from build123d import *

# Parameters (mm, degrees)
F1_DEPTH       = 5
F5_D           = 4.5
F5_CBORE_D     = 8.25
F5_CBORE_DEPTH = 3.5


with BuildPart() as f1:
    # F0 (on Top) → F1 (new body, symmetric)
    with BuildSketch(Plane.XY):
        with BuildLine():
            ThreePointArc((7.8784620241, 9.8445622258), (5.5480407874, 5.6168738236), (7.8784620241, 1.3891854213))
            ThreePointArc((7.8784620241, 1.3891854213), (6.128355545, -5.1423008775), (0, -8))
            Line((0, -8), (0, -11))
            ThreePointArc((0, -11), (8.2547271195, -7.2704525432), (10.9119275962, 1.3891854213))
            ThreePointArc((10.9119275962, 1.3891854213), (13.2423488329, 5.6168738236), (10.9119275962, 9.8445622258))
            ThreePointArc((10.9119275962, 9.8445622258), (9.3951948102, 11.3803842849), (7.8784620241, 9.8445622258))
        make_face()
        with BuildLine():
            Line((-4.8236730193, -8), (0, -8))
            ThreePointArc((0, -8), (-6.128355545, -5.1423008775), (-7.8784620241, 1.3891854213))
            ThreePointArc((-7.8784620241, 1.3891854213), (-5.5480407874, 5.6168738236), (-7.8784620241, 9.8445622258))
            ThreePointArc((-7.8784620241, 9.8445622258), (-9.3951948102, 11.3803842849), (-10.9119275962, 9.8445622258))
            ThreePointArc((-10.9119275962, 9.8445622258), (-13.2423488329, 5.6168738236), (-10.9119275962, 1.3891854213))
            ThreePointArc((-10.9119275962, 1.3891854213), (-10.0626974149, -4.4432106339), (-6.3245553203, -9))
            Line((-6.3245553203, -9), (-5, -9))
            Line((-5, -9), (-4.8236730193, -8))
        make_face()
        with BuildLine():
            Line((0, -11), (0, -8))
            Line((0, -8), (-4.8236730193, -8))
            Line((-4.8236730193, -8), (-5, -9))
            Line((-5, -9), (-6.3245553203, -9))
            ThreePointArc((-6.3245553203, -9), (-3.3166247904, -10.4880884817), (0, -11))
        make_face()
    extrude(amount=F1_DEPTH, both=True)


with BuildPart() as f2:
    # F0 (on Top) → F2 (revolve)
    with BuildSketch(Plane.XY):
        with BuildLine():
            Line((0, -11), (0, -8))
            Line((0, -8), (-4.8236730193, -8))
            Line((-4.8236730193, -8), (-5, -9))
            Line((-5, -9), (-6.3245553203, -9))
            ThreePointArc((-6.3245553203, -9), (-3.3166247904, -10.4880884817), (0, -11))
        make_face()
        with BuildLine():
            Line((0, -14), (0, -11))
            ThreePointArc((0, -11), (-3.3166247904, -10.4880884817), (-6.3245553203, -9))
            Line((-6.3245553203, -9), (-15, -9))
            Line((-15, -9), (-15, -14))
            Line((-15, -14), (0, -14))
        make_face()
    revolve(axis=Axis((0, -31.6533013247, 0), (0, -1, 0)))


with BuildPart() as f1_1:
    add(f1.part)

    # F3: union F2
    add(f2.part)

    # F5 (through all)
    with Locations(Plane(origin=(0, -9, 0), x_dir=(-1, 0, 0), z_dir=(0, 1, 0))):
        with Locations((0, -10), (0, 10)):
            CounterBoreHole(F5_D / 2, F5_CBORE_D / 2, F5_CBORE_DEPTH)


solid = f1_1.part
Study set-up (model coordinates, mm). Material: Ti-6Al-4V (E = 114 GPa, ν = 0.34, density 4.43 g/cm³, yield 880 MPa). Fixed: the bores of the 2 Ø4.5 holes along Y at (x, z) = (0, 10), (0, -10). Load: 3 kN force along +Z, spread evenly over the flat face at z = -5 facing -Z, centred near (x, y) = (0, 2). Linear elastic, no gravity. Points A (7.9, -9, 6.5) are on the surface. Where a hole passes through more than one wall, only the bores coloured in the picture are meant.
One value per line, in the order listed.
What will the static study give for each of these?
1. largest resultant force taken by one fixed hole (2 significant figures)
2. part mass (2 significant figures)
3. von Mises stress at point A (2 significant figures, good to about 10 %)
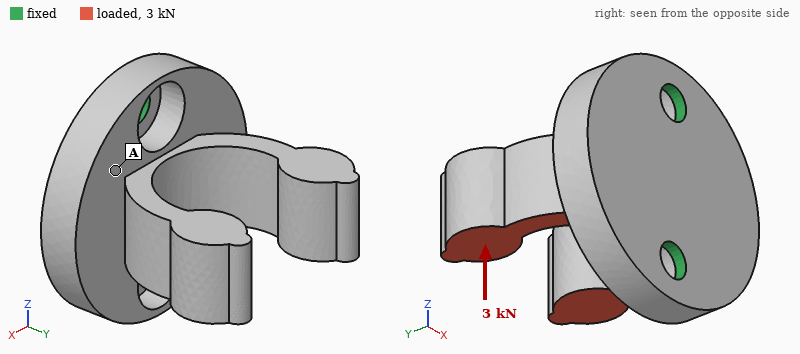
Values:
2.8 kN
22 g
76 MPa
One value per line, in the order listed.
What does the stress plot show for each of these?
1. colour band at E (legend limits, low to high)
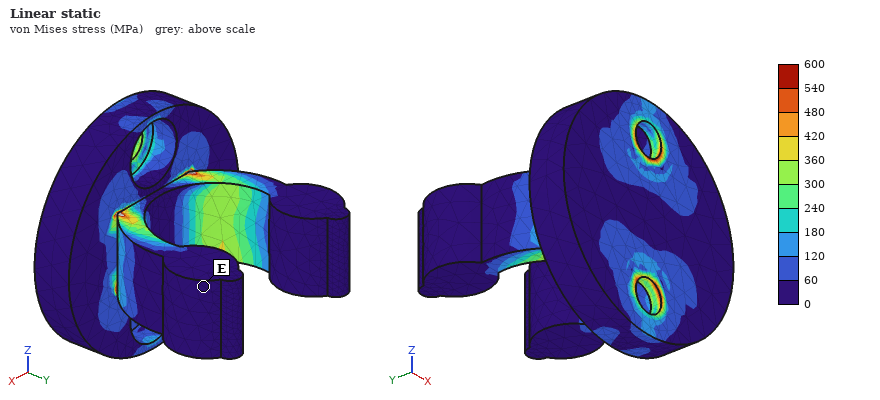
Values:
0 to 60 MPa
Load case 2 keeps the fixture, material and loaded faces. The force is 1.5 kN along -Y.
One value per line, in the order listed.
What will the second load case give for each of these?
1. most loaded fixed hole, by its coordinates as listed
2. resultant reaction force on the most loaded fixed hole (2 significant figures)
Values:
(0, -10)
1.3 kN
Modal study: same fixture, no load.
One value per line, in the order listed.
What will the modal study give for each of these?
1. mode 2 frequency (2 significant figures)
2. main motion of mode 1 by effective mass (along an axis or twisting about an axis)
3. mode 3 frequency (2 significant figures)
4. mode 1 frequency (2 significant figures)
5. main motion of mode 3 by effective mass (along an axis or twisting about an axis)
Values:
4000 Hz
along X
7700 Hz
3000 Hz
along Z
